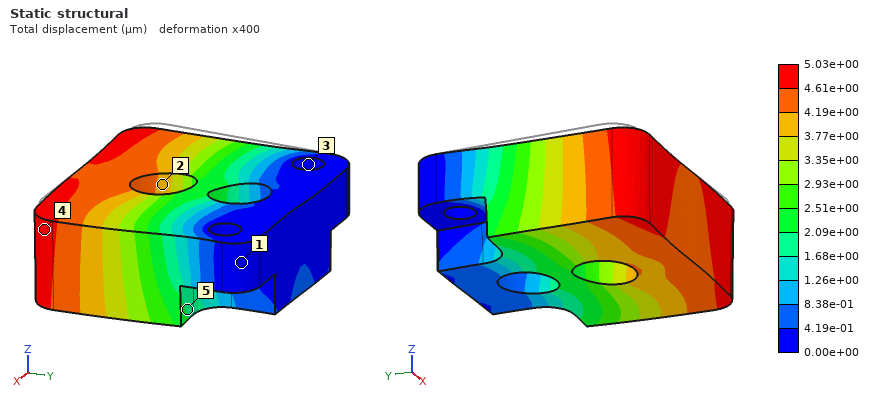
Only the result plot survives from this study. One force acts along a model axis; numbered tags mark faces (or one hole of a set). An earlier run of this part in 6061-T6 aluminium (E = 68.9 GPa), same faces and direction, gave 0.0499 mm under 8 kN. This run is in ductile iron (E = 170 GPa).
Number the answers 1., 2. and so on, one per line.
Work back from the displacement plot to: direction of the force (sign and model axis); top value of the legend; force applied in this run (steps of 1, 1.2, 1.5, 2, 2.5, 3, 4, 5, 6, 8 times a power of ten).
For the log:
1. +X
2. 5.03e+00 µm
3. 2 kN
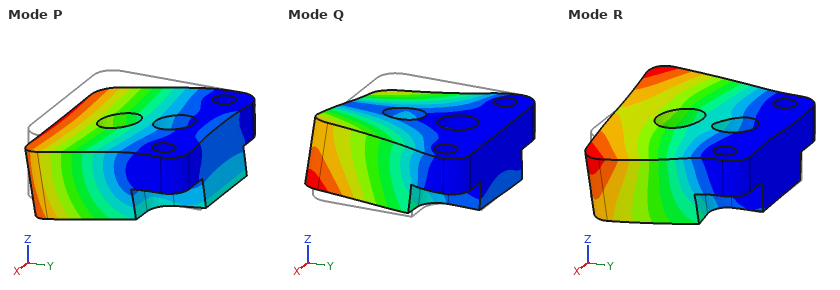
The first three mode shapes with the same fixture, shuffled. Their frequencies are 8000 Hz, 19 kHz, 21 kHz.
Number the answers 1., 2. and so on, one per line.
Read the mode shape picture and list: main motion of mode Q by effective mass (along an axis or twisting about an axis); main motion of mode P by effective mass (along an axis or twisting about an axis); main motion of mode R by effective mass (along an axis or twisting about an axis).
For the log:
1. along X
2. along Z
3. along X
